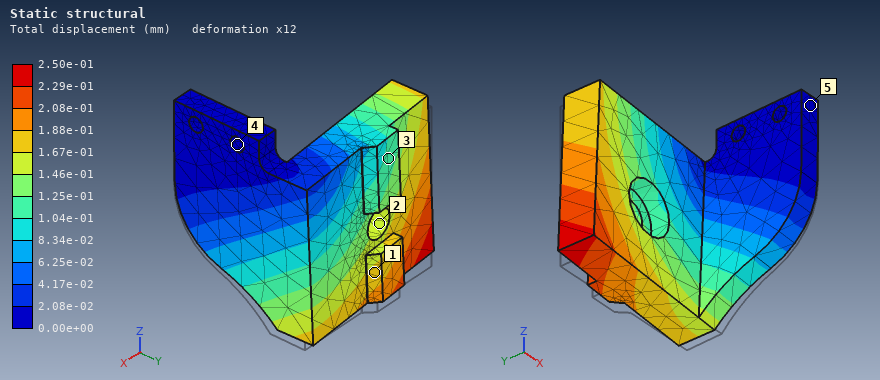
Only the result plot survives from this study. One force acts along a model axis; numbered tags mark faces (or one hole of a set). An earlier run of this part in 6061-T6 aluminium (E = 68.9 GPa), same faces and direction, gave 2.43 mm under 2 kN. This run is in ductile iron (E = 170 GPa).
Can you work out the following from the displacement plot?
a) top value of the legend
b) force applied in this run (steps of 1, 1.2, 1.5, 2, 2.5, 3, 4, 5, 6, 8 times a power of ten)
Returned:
2.50e-01 mm
500 N
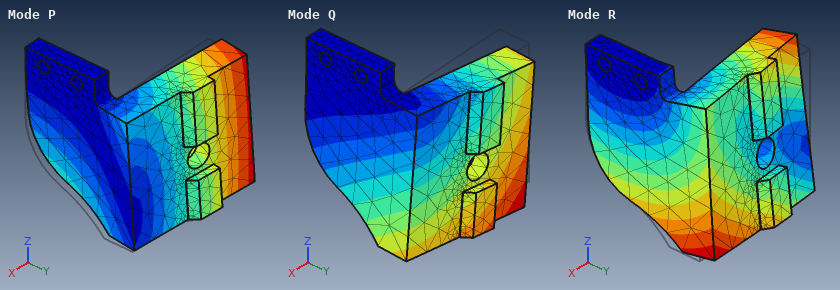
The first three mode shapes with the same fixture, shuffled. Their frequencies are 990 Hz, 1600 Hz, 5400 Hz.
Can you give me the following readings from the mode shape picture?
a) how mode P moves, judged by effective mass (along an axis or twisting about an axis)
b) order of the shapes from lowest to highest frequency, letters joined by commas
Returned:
along Y
Q, P, R
